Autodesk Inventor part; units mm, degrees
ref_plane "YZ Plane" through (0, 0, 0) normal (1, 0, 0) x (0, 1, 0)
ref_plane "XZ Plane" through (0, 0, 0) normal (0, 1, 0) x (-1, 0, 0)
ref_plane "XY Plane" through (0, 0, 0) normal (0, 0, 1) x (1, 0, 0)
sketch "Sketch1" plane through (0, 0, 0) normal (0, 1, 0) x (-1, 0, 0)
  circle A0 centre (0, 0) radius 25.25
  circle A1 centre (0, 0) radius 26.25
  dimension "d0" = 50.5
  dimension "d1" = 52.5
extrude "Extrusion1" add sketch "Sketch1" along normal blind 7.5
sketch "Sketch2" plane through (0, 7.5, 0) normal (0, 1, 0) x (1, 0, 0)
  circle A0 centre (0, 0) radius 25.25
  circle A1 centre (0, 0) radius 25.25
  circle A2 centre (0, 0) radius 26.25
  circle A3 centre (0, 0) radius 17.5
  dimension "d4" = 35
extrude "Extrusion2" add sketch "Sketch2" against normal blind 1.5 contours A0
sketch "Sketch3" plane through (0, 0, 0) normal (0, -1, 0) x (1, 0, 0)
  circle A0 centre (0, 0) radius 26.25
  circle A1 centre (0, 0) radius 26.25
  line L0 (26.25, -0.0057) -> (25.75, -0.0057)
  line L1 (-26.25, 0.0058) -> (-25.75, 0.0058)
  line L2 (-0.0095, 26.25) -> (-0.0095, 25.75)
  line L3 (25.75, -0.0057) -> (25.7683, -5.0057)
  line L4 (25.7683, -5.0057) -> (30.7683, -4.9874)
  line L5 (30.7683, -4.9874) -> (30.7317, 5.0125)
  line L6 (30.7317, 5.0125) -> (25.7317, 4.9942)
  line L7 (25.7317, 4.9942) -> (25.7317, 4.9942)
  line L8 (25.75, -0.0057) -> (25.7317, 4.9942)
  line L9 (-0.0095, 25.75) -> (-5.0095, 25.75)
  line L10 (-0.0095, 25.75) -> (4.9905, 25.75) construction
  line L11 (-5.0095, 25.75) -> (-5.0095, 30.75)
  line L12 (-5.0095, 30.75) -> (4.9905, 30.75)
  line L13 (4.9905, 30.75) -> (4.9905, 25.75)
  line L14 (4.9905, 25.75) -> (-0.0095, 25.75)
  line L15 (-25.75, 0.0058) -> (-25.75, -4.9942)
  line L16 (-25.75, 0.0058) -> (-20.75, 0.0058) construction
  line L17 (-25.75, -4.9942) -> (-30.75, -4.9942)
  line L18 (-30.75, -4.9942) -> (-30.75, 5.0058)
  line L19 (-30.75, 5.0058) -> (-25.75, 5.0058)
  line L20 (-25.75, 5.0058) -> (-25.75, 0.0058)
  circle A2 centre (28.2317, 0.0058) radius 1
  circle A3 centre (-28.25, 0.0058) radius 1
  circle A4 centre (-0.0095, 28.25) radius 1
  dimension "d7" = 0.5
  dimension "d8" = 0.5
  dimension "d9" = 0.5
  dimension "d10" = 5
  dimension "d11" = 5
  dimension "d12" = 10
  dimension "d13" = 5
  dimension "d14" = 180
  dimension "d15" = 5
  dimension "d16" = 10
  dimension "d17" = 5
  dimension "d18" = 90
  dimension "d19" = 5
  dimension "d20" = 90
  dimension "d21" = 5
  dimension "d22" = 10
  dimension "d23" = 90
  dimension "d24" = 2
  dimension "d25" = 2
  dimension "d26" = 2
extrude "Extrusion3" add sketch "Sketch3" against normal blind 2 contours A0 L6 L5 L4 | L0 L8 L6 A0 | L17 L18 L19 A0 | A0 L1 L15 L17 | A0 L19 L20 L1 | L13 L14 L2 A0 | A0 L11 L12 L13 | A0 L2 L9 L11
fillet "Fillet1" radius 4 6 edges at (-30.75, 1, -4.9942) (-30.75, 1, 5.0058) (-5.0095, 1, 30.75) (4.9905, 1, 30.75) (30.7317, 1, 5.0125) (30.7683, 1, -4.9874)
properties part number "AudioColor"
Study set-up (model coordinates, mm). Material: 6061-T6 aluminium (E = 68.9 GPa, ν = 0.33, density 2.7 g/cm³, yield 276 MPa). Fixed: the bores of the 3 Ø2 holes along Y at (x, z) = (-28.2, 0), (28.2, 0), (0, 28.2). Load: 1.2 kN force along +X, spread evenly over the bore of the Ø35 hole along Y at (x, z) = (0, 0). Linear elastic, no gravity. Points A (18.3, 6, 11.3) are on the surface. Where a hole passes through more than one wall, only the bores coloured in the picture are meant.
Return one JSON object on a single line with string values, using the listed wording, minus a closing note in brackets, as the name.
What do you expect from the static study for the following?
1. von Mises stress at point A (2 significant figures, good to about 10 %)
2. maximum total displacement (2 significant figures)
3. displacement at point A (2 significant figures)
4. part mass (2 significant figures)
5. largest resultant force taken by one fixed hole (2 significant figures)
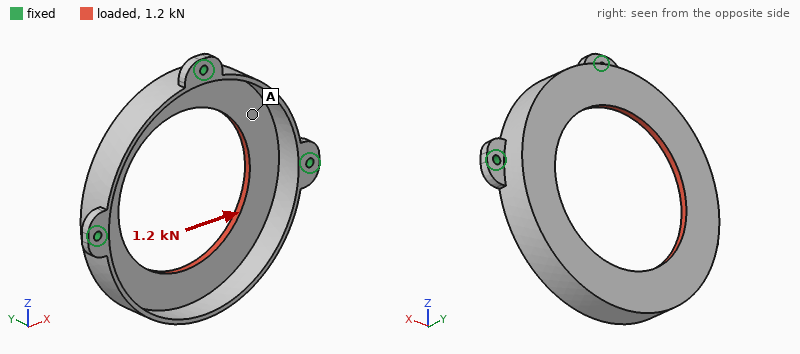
{"von Mises stress at point A": "33 MPa", "maximum total displacement": "0.25 mm", "displacement at point A": "0.044 mm", "part mass": "8.1 g", "largest resultant force taken by one fixed hole": "440 N"}
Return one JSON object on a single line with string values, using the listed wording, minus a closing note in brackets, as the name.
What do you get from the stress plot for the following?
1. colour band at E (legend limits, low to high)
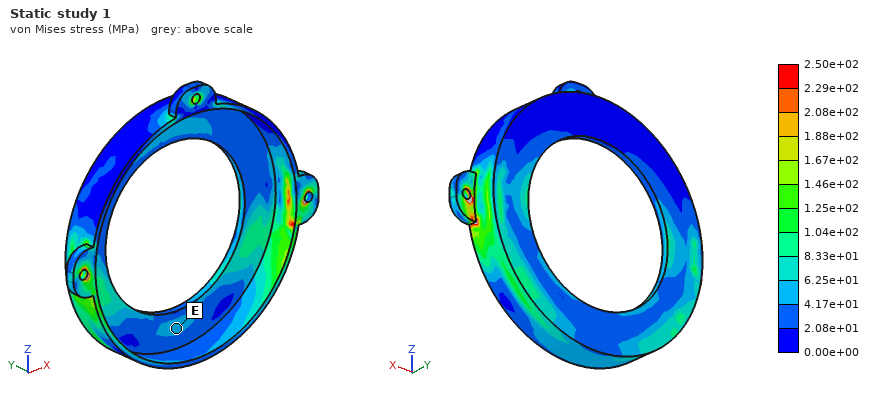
{"colour band at E": "4.17e+01 to 6.25e+01 MPa"}
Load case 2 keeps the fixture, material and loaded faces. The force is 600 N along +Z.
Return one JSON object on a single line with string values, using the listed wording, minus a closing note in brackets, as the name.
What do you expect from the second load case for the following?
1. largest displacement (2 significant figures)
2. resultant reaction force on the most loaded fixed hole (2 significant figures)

{"largest displacement": "85 µm", "resultant reaction force on the most loaded fixed hole": "240 N"}
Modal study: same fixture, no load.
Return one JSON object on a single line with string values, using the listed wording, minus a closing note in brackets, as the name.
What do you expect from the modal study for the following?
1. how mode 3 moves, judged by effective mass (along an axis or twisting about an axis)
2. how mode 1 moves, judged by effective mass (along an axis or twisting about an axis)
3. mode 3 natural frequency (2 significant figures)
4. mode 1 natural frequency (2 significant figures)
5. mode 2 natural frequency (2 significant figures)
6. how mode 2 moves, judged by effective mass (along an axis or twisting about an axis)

{"how mode 3 moves, judged by effective mass": "along Z", "how mode 1 moves, judged by effective mass": "along Y", "mode 3 natural frequency": "9800 Hz", "mode 1 natural frequency": "3100 Hz", "mode 2 natural frequency": "4700 Hz", "how mode 2 moves, judged by effective mass": "along X"}
